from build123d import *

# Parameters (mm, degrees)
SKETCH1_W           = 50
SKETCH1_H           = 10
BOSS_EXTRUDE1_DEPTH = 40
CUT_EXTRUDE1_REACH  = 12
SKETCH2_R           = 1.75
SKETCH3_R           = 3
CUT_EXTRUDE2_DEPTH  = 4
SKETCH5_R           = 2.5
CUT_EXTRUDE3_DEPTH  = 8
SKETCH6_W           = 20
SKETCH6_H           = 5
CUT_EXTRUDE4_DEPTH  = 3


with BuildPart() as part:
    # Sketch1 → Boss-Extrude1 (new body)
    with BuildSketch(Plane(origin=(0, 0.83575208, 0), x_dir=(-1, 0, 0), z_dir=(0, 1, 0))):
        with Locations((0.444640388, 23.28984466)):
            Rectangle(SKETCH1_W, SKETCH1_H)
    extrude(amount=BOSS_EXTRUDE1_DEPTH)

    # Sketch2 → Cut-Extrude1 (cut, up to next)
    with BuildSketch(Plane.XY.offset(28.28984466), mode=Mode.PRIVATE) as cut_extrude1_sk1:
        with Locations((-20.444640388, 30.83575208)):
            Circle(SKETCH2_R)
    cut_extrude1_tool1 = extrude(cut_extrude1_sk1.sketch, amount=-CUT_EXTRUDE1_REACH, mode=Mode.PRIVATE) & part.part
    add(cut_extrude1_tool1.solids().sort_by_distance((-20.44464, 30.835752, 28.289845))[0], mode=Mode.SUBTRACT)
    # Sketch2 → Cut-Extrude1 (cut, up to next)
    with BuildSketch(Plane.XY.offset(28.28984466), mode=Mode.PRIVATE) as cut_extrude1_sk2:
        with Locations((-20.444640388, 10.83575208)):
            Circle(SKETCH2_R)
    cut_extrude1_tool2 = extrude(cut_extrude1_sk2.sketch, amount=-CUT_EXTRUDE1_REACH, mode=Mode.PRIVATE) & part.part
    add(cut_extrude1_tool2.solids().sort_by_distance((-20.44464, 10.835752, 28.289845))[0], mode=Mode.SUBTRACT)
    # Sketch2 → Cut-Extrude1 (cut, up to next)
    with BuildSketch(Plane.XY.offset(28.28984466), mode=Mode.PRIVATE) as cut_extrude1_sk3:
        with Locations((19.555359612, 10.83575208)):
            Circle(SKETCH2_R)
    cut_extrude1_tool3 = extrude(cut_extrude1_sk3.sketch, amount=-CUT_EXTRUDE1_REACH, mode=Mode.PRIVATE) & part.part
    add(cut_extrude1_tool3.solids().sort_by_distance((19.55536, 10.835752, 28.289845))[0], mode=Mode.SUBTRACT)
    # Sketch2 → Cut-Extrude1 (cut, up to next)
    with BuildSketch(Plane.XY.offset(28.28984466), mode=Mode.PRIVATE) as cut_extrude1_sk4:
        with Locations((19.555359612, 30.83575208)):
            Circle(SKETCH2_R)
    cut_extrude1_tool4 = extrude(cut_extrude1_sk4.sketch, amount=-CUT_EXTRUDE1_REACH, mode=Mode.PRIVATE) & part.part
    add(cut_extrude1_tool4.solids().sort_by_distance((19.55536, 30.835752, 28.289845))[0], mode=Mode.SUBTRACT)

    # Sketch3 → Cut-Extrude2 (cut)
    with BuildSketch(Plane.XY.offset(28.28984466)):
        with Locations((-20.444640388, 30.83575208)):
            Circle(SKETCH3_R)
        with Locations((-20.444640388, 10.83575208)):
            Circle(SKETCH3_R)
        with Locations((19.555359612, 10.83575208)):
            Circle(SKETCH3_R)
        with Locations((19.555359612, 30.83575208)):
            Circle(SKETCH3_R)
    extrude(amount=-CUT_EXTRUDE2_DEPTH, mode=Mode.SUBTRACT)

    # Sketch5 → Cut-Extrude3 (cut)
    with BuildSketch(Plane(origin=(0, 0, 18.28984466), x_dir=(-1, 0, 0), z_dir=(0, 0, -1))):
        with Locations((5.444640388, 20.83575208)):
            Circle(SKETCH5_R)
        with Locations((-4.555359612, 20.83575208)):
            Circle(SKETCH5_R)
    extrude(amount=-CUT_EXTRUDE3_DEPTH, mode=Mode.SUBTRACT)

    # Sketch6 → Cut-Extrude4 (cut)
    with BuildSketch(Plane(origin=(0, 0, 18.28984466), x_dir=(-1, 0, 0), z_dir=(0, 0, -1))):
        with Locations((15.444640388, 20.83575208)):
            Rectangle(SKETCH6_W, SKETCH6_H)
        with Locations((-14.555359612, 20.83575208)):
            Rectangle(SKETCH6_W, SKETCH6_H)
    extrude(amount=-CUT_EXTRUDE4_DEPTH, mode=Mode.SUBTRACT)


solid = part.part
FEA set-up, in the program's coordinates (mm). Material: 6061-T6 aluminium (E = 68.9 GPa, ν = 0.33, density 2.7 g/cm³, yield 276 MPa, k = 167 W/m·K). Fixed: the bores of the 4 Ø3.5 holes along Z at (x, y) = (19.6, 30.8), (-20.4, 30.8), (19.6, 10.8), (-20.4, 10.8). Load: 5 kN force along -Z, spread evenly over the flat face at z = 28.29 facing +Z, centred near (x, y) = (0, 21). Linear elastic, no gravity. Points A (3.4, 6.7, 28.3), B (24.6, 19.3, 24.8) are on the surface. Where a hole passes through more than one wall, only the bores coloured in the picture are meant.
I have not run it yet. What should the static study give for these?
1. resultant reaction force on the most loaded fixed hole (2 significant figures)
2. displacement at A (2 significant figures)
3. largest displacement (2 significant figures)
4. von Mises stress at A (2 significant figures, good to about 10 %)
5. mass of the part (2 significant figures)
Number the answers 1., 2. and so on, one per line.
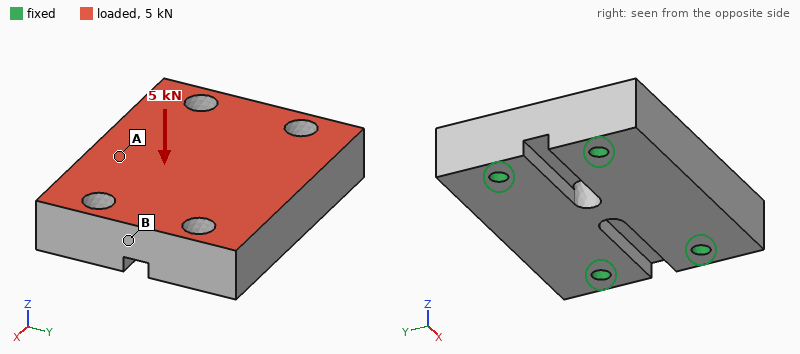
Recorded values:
1. 1.3 kN
2. 10 µm
3. 12 µm
4. 17 MPa
5. 50 g
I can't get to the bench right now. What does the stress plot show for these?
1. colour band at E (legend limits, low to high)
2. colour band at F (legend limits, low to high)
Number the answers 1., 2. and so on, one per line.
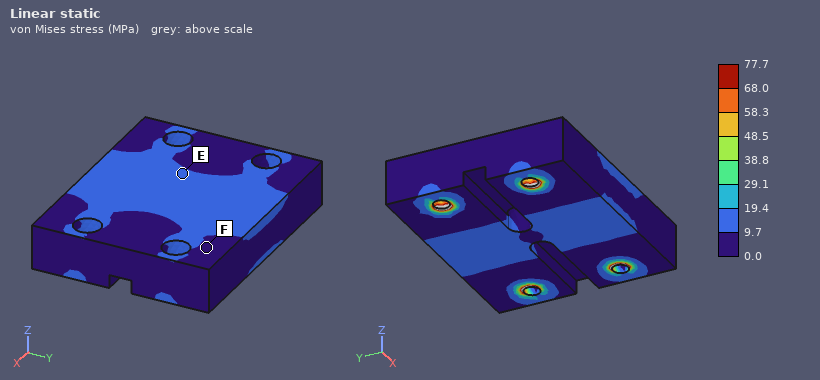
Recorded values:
1. 9.7 to 19.4 MPa
2. 0.0 to 9.7 MPa
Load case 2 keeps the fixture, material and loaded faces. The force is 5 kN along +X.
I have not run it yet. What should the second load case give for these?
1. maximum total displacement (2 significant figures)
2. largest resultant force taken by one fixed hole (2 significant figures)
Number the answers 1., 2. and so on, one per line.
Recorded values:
1. 3.9 µm
2. 1.3 kN
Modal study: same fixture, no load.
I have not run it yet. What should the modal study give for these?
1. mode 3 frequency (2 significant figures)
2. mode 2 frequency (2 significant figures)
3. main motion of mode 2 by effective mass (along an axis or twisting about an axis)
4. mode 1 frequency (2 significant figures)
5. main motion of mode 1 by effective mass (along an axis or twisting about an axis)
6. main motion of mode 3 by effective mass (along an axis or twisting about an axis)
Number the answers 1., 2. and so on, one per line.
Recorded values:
1. 28 kHz
2. 19 kHz
3. twisting about X
4. 17 kHz
5. along Z
6. along Y
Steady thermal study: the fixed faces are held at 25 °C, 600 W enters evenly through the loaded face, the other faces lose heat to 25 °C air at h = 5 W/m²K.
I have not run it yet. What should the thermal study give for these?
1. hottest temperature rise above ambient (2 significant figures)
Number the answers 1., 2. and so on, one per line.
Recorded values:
1. 70 K
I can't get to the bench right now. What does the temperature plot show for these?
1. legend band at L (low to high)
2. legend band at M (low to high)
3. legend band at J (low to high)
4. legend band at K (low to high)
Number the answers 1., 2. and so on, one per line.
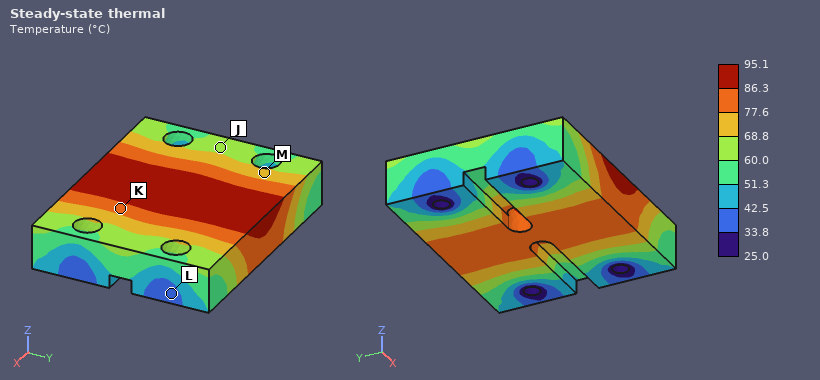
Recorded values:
1. 33.8 to 42.5 °C
2. 68.8 to 77.6 °C
3. 60.0 to 68.8 °C
4. 77.6 to 86.3 °C
